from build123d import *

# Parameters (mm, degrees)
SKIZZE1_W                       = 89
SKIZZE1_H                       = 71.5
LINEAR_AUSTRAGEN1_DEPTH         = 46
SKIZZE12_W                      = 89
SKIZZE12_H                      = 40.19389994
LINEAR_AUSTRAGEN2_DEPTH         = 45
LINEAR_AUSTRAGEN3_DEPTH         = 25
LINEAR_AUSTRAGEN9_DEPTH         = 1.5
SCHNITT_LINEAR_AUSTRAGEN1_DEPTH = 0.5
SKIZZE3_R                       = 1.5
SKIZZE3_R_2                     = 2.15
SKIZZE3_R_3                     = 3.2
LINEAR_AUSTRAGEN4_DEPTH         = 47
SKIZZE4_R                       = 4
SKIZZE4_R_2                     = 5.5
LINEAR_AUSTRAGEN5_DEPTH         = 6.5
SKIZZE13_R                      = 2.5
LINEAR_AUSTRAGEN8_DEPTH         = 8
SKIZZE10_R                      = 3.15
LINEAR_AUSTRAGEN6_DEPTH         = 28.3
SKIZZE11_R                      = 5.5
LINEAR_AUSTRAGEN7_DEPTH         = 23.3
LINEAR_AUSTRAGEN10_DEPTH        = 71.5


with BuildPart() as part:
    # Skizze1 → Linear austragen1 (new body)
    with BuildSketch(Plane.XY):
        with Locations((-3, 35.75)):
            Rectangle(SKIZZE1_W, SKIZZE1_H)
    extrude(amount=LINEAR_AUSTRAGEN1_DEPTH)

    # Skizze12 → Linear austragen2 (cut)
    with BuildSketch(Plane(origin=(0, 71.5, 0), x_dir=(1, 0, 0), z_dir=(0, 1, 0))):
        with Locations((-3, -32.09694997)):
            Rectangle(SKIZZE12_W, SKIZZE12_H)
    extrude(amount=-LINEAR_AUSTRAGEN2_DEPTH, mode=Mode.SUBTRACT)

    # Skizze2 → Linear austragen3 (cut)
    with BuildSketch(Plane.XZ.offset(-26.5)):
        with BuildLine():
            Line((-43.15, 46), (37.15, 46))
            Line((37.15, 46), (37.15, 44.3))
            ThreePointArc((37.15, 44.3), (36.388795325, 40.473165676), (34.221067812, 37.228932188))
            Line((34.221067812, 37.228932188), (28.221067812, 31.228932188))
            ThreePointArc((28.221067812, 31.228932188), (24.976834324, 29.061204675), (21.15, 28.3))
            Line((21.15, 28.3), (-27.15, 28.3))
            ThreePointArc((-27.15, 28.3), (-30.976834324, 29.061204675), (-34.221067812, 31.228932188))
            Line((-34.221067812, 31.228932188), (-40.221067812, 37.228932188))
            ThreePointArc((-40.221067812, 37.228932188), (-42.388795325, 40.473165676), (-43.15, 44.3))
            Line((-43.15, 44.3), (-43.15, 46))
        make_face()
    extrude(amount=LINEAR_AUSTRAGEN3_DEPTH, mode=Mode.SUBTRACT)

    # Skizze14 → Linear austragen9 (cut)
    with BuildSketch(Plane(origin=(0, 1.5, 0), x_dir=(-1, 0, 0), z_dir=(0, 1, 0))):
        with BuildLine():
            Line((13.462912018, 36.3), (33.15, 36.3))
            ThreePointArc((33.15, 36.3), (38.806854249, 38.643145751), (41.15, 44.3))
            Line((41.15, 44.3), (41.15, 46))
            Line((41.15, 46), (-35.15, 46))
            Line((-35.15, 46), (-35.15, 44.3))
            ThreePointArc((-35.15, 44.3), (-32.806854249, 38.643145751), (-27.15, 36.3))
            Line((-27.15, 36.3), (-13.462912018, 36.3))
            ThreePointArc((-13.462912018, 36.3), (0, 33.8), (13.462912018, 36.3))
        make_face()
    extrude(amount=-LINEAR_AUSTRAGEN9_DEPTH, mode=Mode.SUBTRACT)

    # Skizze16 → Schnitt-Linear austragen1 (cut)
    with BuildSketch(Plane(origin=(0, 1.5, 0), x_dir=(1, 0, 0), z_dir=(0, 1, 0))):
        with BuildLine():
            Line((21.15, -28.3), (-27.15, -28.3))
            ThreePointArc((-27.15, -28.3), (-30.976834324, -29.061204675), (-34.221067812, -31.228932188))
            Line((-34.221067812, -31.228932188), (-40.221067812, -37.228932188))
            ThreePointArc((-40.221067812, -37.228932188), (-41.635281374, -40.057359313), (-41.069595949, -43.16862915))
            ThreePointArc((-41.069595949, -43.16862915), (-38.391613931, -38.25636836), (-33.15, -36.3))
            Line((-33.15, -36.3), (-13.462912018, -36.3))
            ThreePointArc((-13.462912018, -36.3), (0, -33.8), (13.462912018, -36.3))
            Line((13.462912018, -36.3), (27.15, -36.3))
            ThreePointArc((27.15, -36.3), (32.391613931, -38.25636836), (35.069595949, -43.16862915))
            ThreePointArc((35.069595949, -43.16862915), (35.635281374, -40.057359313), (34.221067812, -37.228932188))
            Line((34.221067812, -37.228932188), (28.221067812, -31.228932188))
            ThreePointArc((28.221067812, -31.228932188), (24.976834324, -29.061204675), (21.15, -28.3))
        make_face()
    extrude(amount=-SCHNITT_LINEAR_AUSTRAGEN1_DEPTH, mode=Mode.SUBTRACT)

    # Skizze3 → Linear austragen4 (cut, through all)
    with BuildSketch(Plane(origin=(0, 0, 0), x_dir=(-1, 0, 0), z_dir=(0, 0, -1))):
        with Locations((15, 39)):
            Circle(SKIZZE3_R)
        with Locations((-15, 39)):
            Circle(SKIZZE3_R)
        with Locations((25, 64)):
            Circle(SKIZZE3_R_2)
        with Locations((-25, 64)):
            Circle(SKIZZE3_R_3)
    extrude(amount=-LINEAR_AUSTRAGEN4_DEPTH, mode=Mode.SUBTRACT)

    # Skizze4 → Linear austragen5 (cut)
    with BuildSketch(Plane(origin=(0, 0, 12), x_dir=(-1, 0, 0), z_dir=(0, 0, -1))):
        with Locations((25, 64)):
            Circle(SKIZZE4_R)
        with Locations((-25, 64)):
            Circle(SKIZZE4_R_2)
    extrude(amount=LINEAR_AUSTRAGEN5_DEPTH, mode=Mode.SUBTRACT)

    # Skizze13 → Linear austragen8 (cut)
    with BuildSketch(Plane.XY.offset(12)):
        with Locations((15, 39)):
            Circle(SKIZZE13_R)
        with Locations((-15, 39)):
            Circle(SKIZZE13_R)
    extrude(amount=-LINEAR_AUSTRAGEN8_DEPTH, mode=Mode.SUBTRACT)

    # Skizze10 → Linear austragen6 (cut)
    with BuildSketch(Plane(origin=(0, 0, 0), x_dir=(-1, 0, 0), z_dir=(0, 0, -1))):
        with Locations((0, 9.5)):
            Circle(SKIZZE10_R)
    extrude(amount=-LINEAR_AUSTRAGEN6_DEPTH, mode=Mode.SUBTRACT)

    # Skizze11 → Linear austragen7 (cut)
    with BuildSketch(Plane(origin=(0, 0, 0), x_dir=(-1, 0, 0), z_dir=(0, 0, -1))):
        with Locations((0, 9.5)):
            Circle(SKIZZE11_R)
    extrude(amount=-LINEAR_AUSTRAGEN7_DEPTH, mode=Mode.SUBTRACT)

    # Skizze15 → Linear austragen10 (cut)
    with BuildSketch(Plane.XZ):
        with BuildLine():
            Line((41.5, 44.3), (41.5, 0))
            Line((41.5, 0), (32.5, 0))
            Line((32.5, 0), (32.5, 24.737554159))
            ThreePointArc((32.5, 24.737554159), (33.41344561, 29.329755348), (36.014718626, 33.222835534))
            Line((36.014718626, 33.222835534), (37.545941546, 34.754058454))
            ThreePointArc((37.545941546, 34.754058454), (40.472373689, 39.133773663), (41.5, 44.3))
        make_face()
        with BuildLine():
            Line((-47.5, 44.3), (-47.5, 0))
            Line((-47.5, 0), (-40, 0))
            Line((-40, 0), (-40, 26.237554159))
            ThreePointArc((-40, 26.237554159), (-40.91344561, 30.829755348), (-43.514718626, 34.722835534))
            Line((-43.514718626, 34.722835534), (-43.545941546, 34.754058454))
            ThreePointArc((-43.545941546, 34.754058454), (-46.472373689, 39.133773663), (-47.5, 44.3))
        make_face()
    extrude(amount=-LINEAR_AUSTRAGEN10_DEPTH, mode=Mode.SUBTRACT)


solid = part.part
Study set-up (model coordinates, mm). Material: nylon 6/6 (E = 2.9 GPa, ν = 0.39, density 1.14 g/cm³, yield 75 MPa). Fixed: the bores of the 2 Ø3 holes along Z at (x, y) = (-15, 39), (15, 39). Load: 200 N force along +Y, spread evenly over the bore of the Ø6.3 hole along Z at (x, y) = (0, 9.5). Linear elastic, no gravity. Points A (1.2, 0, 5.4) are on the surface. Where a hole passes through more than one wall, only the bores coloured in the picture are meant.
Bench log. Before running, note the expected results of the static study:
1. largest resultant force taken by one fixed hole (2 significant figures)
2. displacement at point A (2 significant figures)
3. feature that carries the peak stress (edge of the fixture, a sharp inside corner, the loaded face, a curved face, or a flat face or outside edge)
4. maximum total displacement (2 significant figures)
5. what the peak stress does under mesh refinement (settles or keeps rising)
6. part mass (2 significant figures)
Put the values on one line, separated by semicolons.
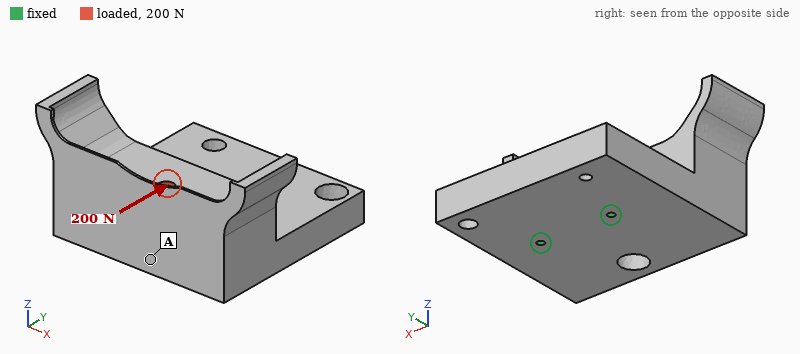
100 N; 0.79 mm; edge of the fixture; 1.2 mm; keeps rising; 110 g
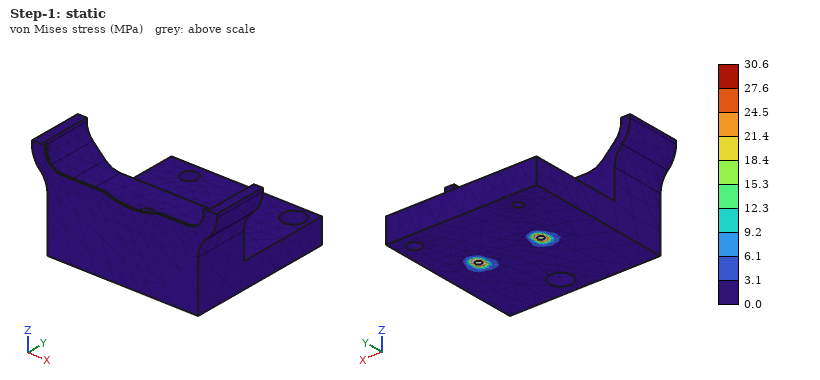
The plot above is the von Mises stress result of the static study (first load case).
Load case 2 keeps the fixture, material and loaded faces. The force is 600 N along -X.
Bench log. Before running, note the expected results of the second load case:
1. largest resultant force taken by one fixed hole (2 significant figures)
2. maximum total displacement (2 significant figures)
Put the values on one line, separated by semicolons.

790 N; 0.31 mm
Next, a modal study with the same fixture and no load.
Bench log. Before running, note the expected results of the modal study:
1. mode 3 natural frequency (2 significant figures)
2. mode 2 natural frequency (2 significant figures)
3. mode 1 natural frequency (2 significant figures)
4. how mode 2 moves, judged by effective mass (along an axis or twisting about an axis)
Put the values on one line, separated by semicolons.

1400 Hz; 1100 Hz; 280 Hz; along X
